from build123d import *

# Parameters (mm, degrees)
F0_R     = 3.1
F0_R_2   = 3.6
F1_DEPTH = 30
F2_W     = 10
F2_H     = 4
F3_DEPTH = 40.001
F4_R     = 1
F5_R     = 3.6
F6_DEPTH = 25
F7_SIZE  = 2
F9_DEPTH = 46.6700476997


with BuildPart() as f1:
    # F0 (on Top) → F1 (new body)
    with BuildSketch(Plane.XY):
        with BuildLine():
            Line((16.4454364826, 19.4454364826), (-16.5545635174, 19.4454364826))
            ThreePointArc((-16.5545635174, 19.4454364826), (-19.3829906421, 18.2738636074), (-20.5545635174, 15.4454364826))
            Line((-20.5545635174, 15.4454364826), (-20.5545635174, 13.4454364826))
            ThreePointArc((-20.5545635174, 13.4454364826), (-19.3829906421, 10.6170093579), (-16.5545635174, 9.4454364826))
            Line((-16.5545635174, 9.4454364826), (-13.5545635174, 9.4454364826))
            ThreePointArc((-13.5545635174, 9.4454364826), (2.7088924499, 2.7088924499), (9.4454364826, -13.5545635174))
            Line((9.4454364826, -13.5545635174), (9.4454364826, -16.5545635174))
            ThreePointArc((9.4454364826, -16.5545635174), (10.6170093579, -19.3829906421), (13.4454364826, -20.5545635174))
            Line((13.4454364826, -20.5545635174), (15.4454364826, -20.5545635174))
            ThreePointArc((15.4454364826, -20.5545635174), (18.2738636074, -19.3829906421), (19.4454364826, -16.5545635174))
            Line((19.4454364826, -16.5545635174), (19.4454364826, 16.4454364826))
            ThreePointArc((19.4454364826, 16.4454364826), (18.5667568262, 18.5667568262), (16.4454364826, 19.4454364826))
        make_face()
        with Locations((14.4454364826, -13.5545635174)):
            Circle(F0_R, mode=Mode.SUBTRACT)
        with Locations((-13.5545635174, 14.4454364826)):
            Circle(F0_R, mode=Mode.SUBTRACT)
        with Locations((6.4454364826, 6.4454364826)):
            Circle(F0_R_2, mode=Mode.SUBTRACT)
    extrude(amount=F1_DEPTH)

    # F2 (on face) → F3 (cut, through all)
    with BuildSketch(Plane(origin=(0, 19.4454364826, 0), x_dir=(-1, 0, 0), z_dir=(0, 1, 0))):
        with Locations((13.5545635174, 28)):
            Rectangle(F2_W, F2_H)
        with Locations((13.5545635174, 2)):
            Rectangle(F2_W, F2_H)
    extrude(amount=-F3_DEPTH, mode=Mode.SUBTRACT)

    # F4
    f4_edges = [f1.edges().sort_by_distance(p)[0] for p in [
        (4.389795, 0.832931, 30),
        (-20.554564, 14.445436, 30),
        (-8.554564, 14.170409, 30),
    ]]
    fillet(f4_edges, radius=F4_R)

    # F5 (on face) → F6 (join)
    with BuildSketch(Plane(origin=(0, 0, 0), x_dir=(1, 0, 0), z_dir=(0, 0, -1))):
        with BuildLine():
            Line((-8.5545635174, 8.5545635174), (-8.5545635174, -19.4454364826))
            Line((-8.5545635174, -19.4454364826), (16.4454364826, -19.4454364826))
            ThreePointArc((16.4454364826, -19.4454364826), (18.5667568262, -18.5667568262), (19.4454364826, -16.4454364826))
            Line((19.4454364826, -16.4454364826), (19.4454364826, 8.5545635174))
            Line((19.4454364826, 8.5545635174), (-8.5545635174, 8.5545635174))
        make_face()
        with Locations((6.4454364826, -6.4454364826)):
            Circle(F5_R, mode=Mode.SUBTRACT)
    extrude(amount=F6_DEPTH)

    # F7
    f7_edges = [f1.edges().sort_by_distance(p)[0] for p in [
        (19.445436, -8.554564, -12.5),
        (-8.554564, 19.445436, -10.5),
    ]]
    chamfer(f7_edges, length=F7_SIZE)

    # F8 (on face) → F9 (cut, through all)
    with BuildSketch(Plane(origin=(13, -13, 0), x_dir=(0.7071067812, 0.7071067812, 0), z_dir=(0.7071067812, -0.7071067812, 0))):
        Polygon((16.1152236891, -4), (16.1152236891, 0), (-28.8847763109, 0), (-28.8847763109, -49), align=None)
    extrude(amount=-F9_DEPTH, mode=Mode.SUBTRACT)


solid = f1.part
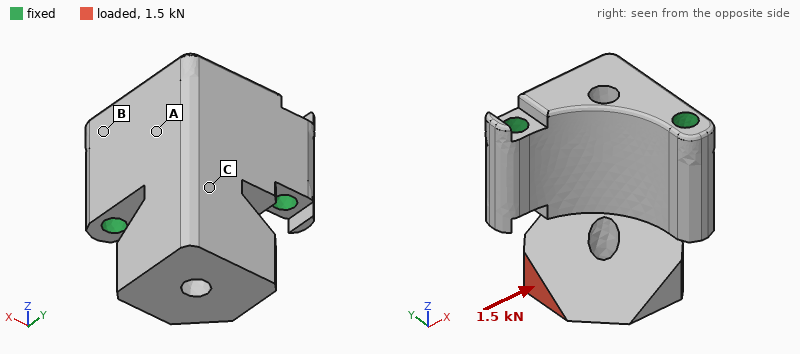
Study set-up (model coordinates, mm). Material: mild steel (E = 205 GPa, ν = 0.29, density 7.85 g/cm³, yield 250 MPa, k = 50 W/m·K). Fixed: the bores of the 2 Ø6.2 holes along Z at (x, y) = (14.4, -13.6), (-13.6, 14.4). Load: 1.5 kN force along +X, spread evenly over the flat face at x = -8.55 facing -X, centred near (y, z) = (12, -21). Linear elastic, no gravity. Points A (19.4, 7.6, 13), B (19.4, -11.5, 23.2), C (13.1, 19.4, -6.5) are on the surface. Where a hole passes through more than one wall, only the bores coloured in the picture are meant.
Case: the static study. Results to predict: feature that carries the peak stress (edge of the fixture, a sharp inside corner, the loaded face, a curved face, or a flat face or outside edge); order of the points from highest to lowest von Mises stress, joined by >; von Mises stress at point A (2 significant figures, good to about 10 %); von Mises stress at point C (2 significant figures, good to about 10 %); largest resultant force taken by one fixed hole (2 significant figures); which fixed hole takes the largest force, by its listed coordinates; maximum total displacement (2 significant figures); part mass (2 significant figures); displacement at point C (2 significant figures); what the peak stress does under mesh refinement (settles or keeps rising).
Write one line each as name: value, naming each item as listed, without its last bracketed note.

feature that carries the peak stress: a sharp inside corner
order of the points from highest to lowest von Mises stress, joined by >: C > A > B
von Mises stress at point A: 25 MPa
von Mises stress at point C: 59 MPa
largest resultant force taken by one fixed hole: 1.7 kN
which fixed hole takes the largest force, by its listed coordinates: (-13.6, 14.4)
maximum total displacement: 72 µm
part mass: 230 g
displacement at point C: 14 µm
what the peak stress does under mesh refinement: keeps rising
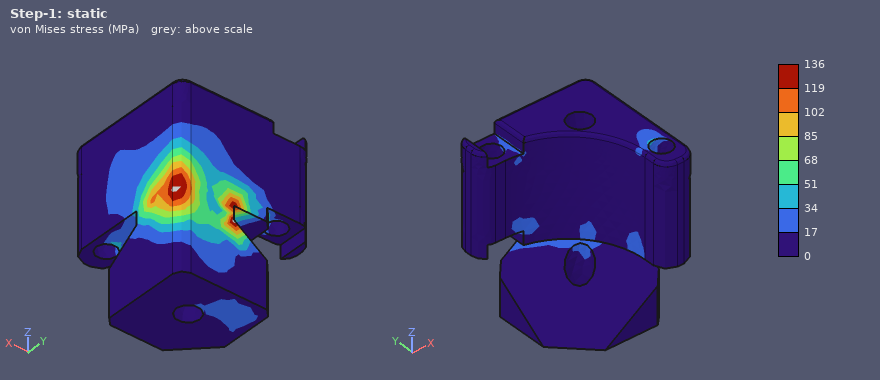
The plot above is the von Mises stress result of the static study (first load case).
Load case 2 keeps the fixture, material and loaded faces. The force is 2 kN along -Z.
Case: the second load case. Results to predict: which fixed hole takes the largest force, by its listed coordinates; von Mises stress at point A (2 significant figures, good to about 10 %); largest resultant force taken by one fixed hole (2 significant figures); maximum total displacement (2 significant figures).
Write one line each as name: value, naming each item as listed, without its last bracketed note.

which fixed hole takes the largest force, by its listed coordinates: (-13.6, 14.4)
von Mises stress at point A: 12 MPa
largest resultant force taken by one fixed hole: 1.7 kN
maximum total displacement: 0.11 mm
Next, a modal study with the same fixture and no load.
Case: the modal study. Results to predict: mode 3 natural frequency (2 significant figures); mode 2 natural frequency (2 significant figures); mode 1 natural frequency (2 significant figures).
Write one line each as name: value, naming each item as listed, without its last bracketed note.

mode 3 natural frequency: 8200 Hz
mode 2 natural frequency: 4300 Hz
mode 1 natural frequency: 3300 Hz
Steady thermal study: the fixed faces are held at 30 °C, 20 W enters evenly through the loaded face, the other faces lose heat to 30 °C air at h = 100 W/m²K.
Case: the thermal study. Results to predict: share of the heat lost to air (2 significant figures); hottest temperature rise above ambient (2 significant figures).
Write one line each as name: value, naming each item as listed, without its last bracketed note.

share of the heat lost to air: 60 %
hottest temperature rise above ambient: 72 K
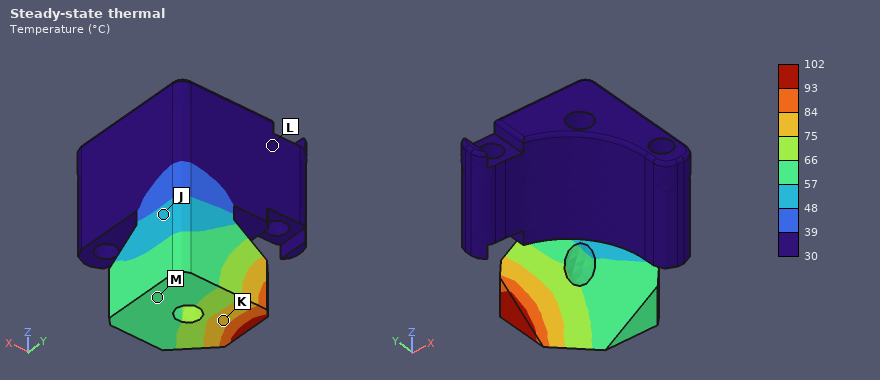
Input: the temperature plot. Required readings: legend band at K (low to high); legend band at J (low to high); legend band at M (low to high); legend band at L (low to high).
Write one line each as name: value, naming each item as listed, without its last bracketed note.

legend band at K: 75 to 84 °C
legend band at J: 48 to 57 °C
legend band at M: 57 to 66 °C
legend band at L: 30 to 39 °C
